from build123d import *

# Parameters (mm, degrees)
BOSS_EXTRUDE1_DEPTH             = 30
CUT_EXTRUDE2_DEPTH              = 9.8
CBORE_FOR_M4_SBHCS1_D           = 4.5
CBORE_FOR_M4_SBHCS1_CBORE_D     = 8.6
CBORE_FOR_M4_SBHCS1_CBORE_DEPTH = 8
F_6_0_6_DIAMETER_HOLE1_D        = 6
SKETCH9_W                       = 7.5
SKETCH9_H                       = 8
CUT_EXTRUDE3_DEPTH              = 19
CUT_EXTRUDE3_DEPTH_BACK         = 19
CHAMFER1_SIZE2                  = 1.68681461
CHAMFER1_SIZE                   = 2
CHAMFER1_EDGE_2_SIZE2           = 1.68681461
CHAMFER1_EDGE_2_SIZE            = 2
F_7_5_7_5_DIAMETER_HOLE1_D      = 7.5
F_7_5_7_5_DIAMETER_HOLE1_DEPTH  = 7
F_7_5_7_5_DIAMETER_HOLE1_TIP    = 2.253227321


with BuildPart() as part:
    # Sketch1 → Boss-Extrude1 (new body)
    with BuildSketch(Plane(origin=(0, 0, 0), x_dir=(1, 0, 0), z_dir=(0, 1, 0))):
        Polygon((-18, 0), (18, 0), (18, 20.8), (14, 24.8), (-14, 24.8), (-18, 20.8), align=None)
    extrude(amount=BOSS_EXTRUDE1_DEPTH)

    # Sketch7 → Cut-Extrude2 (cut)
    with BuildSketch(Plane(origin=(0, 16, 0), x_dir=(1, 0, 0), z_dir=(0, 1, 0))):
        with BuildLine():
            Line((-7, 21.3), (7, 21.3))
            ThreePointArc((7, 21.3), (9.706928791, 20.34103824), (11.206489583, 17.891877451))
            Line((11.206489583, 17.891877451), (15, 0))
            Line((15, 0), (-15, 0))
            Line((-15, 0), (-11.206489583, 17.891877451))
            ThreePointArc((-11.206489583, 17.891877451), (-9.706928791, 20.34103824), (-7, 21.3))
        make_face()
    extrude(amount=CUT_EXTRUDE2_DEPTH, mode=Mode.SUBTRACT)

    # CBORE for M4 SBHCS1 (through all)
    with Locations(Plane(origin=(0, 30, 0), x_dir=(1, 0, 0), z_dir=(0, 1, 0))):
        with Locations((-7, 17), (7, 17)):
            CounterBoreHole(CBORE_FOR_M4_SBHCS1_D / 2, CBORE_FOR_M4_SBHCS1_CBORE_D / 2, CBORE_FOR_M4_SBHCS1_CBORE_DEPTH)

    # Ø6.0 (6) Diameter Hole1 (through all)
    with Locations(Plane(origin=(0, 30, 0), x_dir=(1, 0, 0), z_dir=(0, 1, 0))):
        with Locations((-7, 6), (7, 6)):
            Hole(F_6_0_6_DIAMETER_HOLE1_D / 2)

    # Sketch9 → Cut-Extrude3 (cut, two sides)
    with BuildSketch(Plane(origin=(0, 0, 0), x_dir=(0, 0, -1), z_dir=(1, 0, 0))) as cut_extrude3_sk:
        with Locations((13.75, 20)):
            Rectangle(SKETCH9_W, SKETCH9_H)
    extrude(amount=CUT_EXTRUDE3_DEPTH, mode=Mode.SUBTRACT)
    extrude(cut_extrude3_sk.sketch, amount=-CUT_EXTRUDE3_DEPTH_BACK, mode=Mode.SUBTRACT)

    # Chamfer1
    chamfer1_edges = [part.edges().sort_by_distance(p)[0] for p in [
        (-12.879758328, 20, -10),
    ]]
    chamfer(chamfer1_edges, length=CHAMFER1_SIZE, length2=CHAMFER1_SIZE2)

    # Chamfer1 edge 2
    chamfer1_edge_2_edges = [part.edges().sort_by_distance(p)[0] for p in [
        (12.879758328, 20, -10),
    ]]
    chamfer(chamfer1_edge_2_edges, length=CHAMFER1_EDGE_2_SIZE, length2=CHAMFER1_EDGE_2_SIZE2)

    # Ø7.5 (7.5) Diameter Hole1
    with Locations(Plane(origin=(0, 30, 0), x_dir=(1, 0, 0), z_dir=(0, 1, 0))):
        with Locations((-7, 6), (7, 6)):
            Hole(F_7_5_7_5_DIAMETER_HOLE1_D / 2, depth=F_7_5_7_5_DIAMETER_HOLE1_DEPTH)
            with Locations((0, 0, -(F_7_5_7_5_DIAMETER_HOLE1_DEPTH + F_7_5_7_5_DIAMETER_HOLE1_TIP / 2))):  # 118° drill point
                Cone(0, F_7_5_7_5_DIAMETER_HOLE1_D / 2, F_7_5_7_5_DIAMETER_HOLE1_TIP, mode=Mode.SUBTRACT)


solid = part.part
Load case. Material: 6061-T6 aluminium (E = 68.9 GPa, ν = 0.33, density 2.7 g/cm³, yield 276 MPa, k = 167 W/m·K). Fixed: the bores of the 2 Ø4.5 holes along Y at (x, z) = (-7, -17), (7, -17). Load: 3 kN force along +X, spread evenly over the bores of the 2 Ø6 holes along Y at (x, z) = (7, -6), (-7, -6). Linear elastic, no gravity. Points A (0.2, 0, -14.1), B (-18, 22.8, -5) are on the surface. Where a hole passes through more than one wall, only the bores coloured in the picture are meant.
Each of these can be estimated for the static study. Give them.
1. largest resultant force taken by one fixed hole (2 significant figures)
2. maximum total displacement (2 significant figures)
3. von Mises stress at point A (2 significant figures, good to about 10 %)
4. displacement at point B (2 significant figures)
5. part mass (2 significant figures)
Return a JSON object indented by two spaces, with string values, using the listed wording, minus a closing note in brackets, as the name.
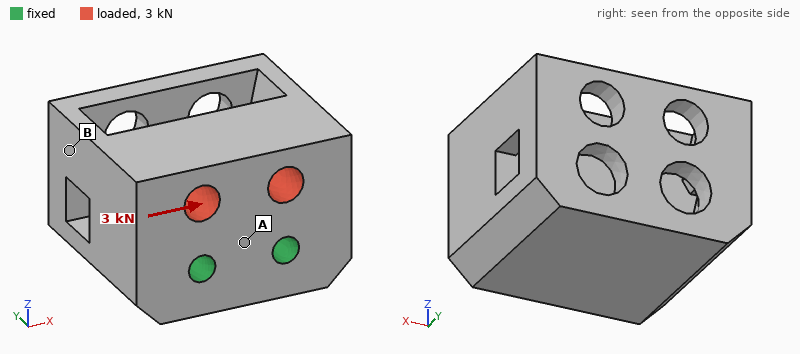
{
  "largest resultant force taken by one fixed hole": "2.2 kN",
  "maximum total displacement": "7.2 µm",
  "von Mises stress at point A": "10 MPa",
  "displacement at point B": "4.9 µm",
  "part mass": "49 g"
}
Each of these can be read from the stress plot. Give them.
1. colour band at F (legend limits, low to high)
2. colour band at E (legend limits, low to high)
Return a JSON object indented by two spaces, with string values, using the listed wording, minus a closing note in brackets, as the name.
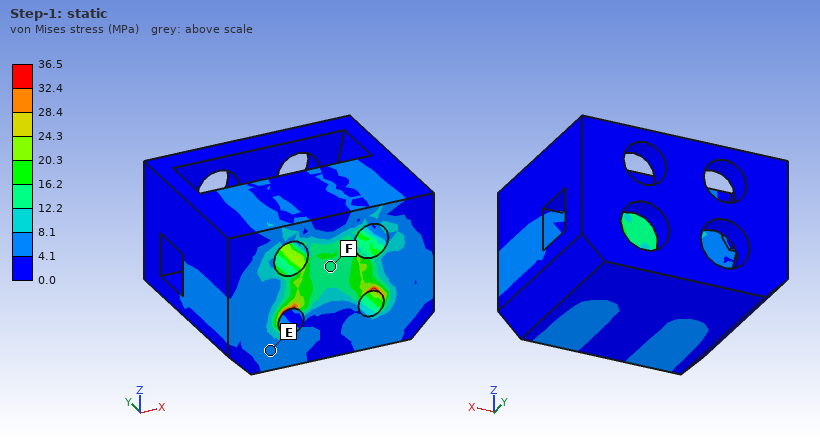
{
  "colour band at F": "12.2 to 16.2 MPa",
  "colour band at E": "4.1 to 8.1 MPa"
}
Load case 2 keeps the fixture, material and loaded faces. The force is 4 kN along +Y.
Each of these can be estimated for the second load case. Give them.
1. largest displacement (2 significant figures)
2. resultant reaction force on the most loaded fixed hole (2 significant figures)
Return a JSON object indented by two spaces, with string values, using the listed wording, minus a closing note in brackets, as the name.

{
  "largest displacement": "10 µm",
  "resultant reaction force on the most loaded fixed hole": "2.0 kN"
}
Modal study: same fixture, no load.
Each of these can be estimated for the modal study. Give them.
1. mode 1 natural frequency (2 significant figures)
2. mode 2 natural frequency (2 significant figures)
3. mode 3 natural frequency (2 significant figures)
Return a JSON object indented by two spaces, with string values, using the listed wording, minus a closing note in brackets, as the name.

{
  "mode 1 natural frequency": "12 kHz",
  "mode 2 natural frequency": "13 kHz",
  "mode 3 natural frequency": "18 kHz"
}
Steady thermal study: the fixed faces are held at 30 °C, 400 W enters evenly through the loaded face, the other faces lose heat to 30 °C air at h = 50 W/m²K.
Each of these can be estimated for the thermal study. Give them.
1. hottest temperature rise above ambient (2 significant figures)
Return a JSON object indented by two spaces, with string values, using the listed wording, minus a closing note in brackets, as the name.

{
  "hottest temperature rise above ambient": "65 K"
}
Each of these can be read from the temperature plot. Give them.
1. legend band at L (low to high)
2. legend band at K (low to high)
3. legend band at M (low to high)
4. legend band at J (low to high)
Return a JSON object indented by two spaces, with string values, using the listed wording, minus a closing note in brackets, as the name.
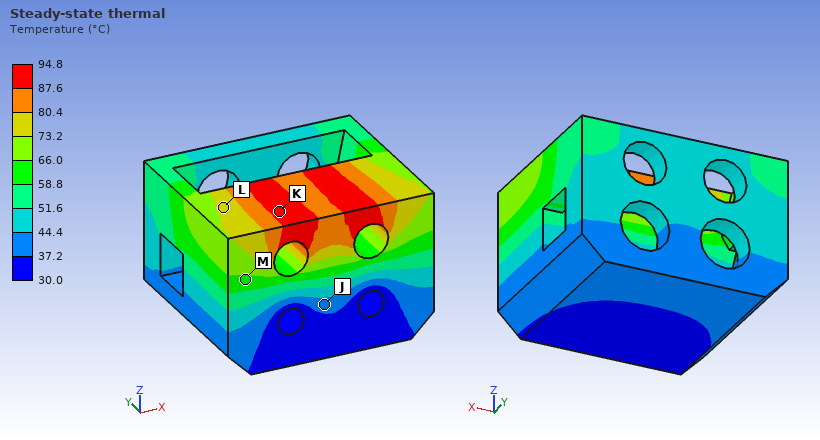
{
  "legend band at L": "73.2 to 80.4 °C",
  "legend band at K": "87.6 to 94.8 °C",
  "legend band at M": "58.8 to 66.0 °C",
  "legend band at J": "37.2 to 44.4 °C"
}
